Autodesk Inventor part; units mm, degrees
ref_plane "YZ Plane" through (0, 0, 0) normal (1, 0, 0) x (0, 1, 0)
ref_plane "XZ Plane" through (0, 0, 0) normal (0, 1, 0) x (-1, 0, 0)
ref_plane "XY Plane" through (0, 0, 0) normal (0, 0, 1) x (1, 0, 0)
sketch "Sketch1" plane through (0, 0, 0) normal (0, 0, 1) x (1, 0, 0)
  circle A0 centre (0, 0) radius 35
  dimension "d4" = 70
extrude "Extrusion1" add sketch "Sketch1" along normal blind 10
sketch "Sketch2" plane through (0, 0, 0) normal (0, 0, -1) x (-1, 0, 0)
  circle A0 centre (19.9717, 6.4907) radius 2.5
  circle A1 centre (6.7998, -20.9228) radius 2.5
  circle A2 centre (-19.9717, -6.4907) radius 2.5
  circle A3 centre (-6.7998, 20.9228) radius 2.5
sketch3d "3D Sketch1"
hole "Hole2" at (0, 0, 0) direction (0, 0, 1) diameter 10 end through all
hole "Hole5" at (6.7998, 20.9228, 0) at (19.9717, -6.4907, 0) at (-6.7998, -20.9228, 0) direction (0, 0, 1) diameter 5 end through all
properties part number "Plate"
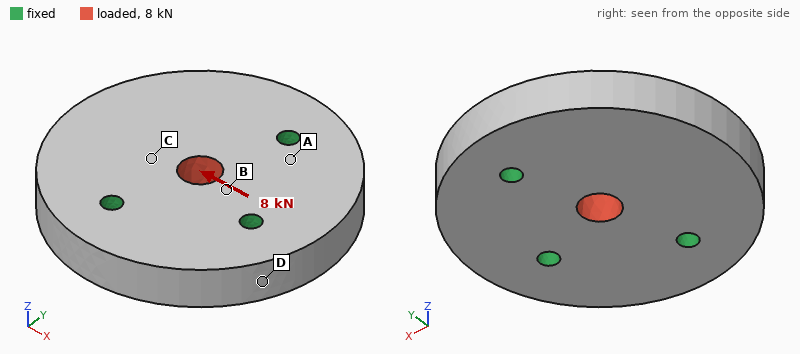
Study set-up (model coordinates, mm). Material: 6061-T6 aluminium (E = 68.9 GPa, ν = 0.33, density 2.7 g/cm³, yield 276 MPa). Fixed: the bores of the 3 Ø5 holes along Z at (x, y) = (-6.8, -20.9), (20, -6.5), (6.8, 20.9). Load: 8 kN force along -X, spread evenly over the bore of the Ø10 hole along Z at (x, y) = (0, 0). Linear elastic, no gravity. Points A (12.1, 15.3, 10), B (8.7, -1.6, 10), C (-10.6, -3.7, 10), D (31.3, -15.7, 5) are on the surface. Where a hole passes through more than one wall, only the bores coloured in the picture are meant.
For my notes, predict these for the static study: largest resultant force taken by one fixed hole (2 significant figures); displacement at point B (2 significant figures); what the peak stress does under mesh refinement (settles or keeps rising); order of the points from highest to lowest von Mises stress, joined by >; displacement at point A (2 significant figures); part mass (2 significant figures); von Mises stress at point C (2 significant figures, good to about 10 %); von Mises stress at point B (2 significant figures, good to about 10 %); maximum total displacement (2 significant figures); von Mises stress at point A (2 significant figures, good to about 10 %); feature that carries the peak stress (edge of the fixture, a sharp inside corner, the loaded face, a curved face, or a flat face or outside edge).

3.2 kN
4.2 µm
keeps rising
B > C > A > D
2.0 µm
100 g
17 MPa
27 MPa
8.0 µm
11 MPa
edge of the fixture
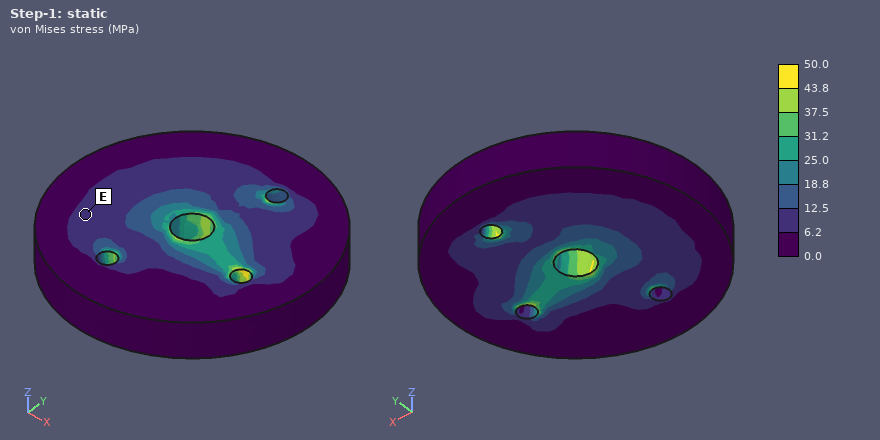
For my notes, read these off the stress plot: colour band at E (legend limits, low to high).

6.2 to 12.5 MPa
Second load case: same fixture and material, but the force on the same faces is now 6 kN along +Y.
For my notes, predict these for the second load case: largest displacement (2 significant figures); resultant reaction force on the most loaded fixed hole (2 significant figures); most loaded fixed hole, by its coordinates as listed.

5.2 µm
2.7 kN
(-6.8, -20.9)
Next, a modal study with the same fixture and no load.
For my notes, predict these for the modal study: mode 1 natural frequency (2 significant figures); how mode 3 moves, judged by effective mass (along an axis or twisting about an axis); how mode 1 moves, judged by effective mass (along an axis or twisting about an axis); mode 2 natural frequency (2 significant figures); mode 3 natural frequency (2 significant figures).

6700 Hz
twisting about X
along Z
14 kHz
18 kHz
